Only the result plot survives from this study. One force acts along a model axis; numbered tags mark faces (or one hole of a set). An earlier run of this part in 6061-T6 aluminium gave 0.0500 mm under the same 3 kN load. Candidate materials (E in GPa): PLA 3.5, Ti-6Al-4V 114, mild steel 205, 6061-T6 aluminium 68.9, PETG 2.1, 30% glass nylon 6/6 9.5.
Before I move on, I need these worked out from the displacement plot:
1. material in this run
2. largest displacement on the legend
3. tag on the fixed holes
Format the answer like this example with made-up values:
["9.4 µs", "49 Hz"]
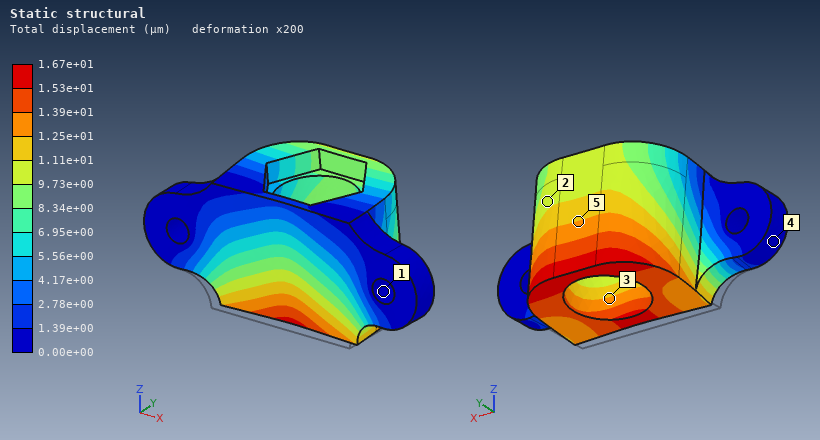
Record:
["mild steel", "1.67e+01 µm", "1"]
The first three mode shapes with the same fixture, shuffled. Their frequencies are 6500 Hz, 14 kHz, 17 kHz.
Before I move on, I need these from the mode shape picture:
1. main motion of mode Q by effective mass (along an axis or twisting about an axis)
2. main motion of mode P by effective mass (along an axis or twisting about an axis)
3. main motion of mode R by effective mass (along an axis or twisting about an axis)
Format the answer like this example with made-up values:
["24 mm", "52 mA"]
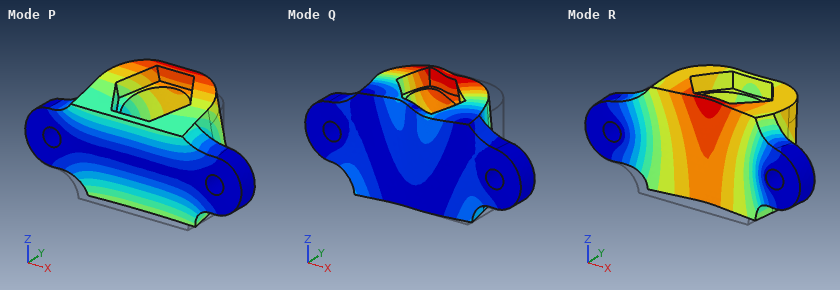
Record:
["along X", "along Z", "along Y"]
